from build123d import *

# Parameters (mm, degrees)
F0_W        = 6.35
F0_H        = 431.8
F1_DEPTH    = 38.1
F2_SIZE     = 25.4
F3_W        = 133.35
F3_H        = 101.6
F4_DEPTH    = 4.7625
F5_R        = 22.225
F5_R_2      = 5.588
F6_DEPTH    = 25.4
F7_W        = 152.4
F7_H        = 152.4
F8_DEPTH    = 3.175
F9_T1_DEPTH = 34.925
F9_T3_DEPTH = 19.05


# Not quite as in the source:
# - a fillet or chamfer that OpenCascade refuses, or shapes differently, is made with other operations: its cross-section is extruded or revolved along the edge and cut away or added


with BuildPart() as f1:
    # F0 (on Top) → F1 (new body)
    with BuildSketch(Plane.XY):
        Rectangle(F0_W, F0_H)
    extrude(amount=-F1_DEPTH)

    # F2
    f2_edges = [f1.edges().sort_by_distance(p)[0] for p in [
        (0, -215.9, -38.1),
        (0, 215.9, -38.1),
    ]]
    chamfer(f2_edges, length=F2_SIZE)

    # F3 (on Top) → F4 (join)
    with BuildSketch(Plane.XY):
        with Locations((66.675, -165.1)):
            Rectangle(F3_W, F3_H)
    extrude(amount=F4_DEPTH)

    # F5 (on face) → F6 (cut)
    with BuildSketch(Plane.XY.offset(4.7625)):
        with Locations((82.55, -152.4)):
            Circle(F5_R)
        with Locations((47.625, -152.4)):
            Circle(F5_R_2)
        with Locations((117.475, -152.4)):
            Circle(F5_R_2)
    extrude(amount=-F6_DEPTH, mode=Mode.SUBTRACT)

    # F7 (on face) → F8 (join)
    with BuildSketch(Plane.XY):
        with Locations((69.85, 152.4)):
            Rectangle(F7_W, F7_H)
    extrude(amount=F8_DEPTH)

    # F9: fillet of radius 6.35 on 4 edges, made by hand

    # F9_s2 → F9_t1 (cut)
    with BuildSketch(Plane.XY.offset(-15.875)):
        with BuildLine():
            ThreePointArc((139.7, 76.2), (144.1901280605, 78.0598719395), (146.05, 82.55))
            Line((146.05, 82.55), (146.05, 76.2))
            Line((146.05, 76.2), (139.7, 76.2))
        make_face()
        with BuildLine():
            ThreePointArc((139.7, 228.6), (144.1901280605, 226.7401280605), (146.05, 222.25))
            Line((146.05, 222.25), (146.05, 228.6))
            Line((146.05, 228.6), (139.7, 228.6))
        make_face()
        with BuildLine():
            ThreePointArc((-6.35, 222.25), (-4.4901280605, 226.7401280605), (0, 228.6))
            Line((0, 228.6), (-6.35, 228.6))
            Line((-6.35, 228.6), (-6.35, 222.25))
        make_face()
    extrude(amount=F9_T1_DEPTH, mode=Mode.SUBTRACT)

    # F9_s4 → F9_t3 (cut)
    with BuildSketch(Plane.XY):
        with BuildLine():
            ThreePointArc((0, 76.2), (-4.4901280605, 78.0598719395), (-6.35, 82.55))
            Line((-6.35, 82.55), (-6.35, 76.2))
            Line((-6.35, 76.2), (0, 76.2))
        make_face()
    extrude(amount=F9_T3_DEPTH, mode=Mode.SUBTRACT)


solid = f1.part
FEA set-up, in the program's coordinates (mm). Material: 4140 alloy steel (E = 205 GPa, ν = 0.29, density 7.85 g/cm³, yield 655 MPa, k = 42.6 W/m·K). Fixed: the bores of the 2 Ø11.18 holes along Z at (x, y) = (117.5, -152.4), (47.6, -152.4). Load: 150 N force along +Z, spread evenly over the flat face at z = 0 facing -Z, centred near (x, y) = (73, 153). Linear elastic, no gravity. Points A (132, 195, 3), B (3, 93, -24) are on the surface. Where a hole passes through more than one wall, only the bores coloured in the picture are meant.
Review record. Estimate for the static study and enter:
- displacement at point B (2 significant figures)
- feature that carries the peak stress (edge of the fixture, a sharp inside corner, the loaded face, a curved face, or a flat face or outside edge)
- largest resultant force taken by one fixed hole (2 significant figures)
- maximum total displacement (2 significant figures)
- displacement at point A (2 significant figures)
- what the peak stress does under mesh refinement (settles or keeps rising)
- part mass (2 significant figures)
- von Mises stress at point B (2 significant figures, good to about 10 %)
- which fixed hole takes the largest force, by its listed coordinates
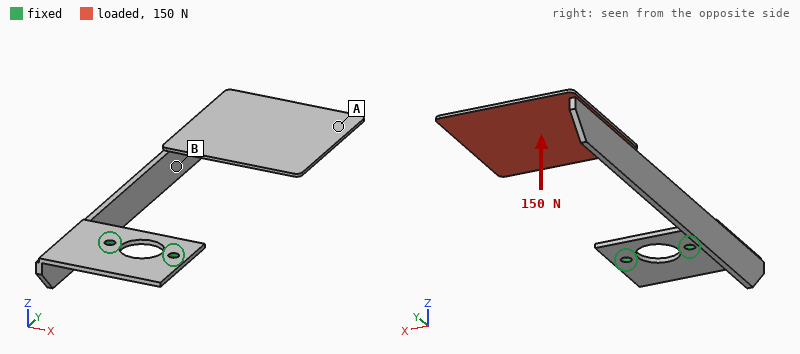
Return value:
1.8 mm
edge of the fixture
130 N
5.4 mm
4.9 mm
keeps rising
1.8 kg
32 MPa
(47.6, -152.4)
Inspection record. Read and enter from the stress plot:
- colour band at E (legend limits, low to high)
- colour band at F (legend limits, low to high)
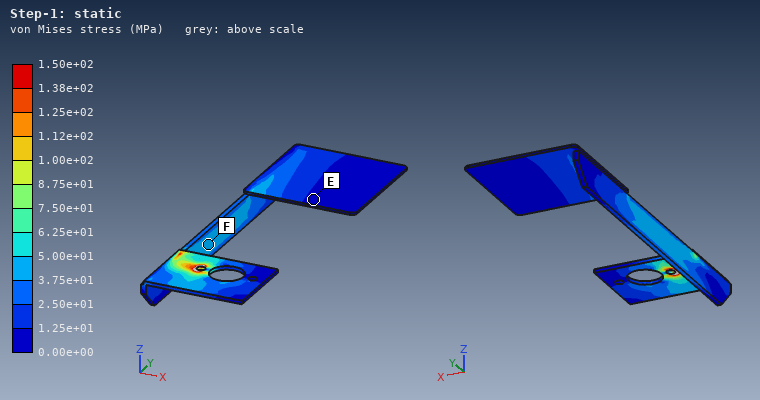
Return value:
0.00e+00 to 1.25e+01 MPa
3.75e+01 to 5.00e+01 MPa
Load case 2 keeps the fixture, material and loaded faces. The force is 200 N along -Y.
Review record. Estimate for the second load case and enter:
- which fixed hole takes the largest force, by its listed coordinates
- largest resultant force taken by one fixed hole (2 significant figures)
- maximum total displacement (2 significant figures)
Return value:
(47.6, -152.4)
150 N
5.6 mm
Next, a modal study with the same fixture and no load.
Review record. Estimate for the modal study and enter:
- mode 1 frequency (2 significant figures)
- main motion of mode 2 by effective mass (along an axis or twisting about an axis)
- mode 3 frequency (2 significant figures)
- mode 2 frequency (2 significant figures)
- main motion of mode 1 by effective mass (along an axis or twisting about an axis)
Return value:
24 Hz
along Z
85 Hz
39 Hz
along X
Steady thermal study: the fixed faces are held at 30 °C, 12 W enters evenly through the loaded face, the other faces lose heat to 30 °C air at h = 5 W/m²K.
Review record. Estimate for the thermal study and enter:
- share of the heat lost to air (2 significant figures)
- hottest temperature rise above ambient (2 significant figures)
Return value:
93 %
62 K
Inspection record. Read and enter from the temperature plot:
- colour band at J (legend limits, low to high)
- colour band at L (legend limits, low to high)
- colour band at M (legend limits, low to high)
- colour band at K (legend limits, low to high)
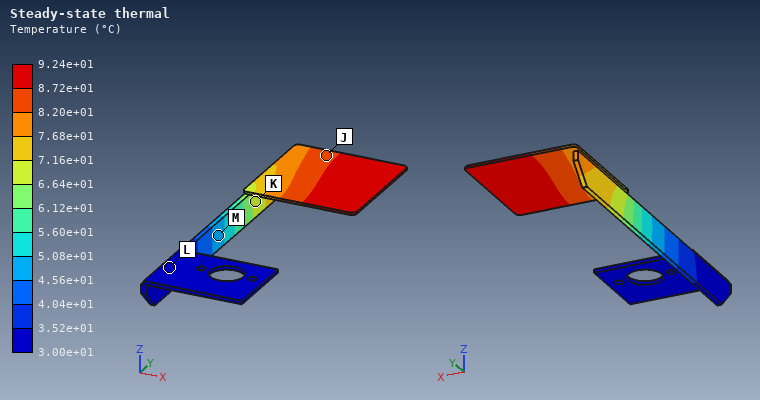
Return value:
8.20e+01 to 8.72e+01 °C
3.00e+01 to 3.52e+01 °C
4.56e+01 to 5.08e+01 °C
6.64e+01 to 7.16e+01 °C
